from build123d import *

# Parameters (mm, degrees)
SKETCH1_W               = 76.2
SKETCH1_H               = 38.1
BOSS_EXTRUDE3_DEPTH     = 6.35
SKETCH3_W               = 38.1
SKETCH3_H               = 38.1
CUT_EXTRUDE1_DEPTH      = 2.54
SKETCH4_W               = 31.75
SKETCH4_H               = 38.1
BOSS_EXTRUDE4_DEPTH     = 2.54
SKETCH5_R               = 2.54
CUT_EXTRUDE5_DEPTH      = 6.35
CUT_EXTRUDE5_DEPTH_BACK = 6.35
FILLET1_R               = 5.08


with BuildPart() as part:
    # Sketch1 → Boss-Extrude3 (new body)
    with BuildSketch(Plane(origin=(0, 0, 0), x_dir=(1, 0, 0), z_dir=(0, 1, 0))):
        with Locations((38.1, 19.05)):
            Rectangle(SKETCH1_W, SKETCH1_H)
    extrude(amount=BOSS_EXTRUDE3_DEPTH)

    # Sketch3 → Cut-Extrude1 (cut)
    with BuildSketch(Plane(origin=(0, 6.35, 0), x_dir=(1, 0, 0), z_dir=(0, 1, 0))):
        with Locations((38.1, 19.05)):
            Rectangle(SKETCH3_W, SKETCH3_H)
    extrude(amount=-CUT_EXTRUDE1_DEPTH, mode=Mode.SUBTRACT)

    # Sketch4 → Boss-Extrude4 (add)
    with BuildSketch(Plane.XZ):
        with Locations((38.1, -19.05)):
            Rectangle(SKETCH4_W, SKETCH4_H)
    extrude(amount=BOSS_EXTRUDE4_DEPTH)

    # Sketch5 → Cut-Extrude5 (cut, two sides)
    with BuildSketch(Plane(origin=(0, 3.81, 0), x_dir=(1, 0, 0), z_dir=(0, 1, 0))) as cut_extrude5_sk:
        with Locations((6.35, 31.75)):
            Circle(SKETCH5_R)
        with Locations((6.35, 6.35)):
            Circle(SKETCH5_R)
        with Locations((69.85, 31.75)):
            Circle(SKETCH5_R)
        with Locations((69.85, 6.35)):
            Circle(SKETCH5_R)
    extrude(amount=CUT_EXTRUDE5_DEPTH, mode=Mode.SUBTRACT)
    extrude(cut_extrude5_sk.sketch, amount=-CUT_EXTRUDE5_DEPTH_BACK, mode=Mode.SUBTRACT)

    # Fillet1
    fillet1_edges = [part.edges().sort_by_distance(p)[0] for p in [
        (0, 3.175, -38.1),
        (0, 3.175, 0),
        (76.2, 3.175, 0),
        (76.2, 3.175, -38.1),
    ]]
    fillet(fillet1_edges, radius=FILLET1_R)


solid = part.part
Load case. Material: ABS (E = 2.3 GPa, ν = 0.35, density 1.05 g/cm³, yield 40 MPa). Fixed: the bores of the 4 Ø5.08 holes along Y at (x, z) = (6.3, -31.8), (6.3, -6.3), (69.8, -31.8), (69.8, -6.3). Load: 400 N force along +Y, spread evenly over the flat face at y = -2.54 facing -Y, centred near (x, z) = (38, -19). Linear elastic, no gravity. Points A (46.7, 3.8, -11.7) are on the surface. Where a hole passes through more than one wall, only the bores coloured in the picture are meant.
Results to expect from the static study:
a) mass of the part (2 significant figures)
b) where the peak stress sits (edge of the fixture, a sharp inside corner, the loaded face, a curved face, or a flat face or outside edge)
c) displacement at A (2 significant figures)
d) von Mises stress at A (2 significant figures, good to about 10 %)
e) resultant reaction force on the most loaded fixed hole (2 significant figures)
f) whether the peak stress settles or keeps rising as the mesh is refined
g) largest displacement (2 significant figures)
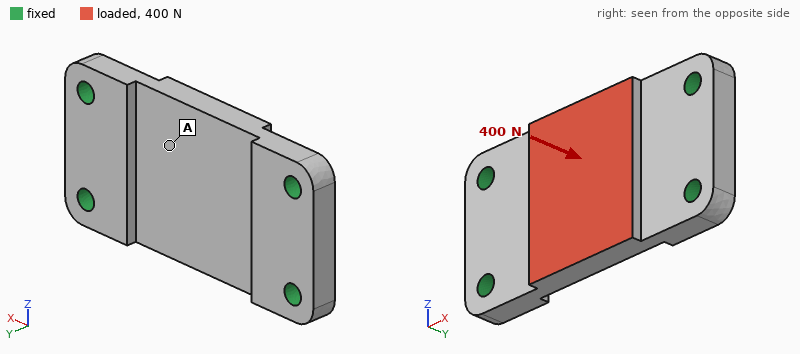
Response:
18 g
edge of the fixture
0.18 mm
2.6 MPa
180 N
keeps rising
0.22 mm
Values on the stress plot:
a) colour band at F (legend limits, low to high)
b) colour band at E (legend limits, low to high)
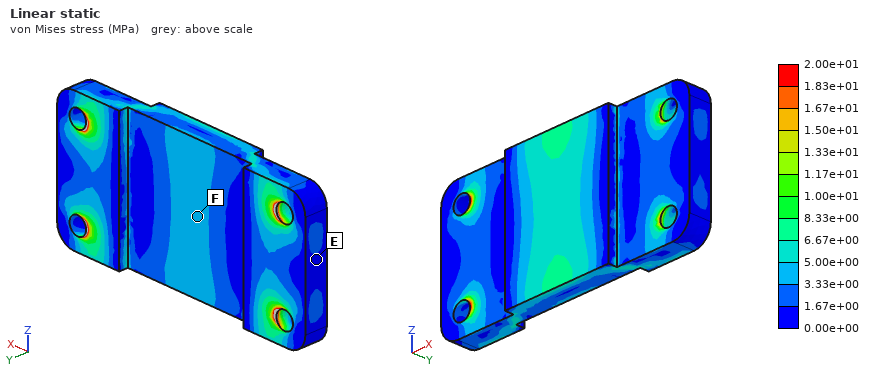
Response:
3.33e+00 to 5.00e+00 MPa
0.00e+00 to 1.67e+00 MPa
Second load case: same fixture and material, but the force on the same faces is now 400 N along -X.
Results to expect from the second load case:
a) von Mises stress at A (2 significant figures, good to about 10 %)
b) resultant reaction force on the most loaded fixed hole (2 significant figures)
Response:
0.62 MPa
100 N
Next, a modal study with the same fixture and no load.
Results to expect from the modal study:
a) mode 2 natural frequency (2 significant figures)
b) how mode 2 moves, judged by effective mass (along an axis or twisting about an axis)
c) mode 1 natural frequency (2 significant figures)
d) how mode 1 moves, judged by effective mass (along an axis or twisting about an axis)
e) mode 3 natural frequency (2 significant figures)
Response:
3200 Hz
twisting about X
2500 Hz
along Y
5100 Hz
